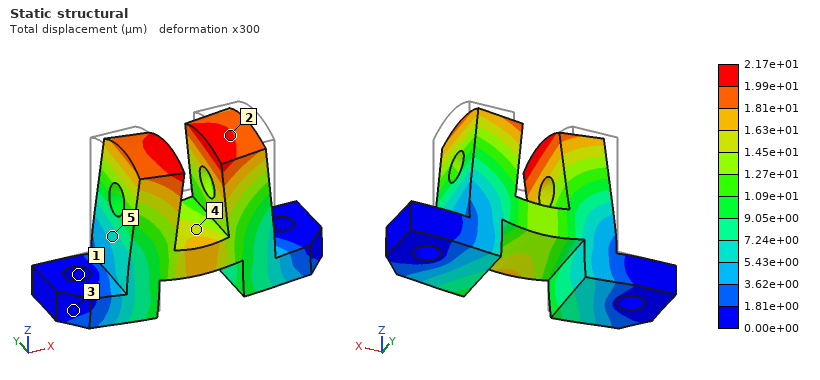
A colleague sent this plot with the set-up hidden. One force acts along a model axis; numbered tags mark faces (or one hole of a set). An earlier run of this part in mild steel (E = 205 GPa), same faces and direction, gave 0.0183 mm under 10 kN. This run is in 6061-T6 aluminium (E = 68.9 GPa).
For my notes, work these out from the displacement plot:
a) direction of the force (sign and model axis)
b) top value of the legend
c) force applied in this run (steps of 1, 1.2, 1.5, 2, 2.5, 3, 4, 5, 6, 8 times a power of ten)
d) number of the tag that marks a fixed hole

-Z
2.17e+01 µm
4 kN
1
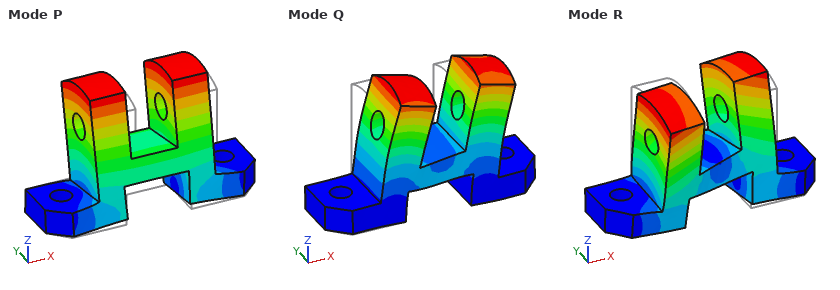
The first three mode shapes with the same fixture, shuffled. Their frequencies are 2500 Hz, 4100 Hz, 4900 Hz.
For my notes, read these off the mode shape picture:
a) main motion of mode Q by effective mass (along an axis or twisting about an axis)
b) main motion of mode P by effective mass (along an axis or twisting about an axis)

along X
along Y
